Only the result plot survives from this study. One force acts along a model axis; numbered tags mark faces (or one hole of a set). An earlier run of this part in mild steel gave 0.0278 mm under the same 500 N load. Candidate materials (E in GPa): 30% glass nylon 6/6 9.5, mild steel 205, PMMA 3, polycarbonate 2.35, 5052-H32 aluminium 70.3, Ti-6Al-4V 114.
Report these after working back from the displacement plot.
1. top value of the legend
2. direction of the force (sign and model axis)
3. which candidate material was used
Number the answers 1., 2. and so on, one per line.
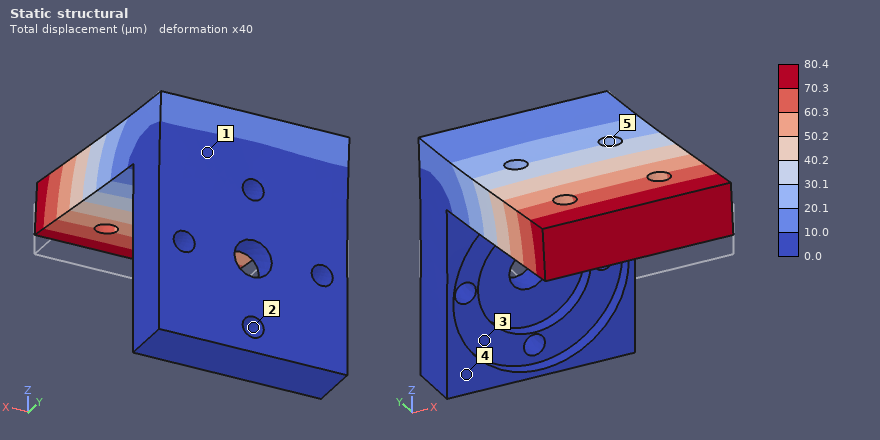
1. 80.4 µm
2. +Z
3. 5052-H32 aluminium
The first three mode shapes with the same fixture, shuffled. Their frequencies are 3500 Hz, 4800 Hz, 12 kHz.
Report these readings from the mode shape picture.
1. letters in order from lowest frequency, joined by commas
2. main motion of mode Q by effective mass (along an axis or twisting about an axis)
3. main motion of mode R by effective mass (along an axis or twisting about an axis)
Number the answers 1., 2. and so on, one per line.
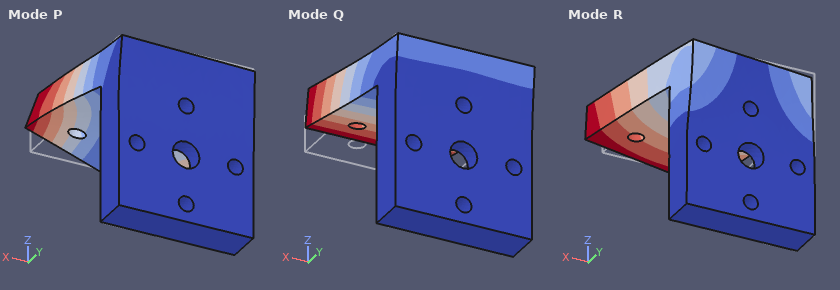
1. Q, R, P
2. along Z
3. along X
